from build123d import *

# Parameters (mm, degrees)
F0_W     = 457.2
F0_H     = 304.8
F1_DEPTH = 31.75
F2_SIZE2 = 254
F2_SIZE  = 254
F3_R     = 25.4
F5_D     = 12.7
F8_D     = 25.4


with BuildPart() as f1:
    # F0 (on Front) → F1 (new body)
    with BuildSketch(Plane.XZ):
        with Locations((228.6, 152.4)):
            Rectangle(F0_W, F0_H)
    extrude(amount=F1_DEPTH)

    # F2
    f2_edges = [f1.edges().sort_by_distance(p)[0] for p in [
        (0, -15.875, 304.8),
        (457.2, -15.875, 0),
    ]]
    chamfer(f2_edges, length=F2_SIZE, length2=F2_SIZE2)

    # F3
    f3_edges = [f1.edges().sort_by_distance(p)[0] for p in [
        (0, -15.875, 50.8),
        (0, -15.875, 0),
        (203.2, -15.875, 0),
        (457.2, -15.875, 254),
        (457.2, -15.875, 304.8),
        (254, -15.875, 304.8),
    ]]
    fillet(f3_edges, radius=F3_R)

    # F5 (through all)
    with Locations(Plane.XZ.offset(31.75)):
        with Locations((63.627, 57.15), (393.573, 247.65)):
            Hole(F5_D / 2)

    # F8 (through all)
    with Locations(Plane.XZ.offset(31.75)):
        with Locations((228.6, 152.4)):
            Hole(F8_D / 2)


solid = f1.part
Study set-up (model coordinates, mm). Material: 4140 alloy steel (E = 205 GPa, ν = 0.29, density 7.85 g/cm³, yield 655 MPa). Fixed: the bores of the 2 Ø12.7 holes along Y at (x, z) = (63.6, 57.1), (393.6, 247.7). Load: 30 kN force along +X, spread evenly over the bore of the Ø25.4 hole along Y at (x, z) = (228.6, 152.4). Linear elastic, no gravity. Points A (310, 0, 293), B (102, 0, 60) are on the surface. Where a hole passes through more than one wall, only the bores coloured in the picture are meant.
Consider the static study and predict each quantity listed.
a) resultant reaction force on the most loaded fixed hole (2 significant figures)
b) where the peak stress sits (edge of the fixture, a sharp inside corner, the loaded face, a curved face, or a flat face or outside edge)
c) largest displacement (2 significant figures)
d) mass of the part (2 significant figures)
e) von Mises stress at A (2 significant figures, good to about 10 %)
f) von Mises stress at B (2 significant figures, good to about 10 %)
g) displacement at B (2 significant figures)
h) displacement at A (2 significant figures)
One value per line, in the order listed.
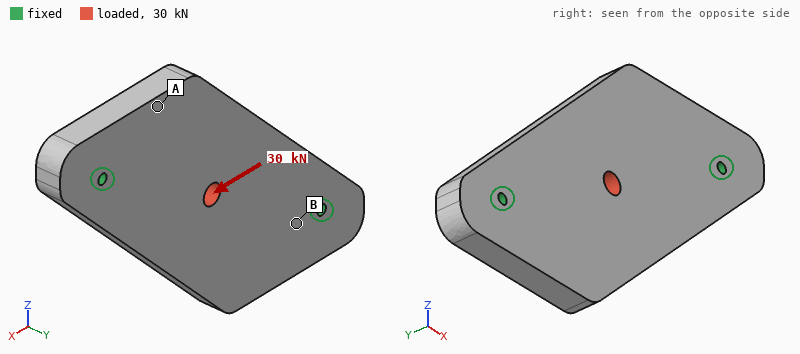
15 kN
edge of the fixture
11 µm
18 kg
3.2 MPa
6.9 MPa
2.2 µm
3.0 µm
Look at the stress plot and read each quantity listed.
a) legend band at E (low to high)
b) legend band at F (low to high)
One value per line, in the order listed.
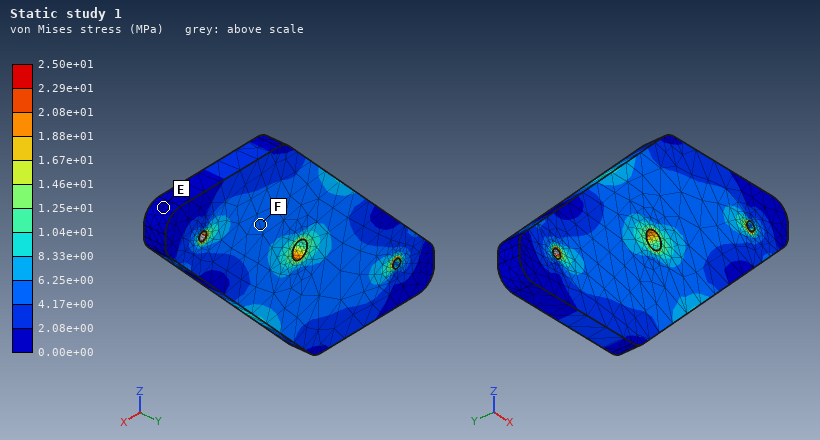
0.00e+00 to 2.08e+00 MPa
4.17e+00 to 6.25e+00 MPa
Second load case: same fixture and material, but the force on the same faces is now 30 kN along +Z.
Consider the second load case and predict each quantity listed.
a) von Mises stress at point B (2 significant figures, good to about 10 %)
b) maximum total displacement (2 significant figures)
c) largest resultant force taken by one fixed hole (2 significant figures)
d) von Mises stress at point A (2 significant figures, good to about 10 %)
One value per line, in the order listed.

6.2 MPa
18 µm
15 kN
4.3 MPa
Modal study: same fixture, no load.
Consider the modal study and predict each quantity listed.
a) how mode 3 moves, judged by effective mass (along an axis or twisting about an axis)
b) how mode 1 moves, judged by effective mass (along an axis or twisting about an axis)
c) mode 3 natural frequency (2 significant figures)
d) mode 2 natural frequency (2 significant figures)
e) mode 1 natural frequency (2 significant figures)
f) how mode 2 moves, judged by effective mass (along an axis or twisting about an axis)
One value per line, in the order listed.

along Z
along Y
2100 Hz
990 Hz
820 Hz
twisting about X
